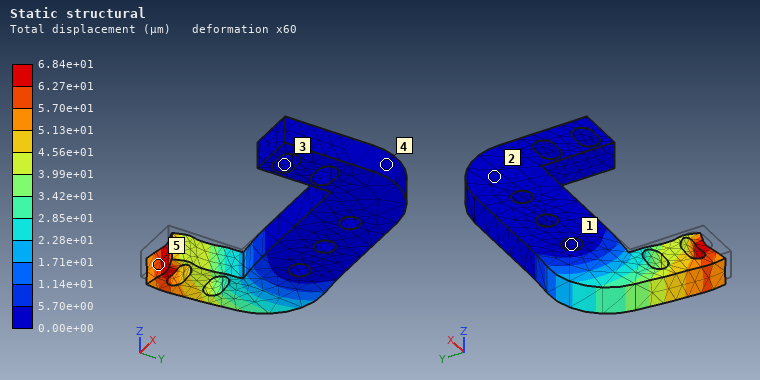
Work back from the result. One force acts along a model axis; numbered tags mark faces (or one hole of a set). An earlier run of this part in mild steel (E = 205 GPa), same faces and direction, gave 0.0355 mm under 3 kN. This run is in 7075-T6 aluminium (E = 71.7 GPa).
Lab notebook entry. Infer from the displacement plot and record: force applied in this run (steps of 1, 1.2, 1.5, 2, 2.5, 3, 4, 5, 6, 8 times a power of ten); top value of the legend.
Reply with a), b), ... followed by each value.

a) 2 kN
b) 6.84e+01 µm
